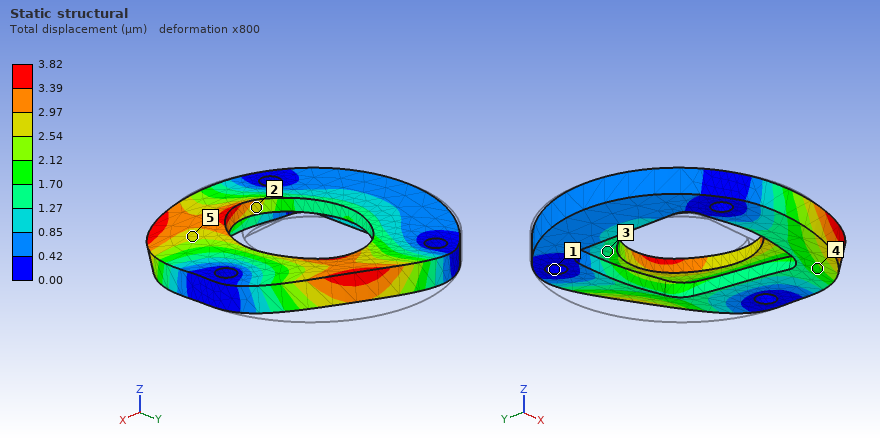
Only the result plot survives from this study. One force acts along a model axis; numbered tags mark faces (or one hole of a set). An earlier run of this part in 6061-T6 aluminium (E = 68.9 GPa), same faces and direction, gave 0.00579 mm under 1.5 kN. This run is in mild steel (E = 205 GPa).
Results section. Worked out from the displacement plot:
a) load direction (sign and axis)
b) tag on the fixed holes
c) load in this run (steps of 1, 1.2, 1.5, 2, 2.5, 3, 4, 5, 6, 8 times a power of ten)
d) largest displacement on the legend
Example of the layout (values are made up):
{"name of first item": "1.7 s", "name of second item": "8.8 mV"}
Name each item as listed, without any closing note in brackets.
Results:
{"load direction": "-Y", "tag on the fixed holes": "1", "load in this run": "3 kN", "largest displacement on the legend": "3.82 µm"}
